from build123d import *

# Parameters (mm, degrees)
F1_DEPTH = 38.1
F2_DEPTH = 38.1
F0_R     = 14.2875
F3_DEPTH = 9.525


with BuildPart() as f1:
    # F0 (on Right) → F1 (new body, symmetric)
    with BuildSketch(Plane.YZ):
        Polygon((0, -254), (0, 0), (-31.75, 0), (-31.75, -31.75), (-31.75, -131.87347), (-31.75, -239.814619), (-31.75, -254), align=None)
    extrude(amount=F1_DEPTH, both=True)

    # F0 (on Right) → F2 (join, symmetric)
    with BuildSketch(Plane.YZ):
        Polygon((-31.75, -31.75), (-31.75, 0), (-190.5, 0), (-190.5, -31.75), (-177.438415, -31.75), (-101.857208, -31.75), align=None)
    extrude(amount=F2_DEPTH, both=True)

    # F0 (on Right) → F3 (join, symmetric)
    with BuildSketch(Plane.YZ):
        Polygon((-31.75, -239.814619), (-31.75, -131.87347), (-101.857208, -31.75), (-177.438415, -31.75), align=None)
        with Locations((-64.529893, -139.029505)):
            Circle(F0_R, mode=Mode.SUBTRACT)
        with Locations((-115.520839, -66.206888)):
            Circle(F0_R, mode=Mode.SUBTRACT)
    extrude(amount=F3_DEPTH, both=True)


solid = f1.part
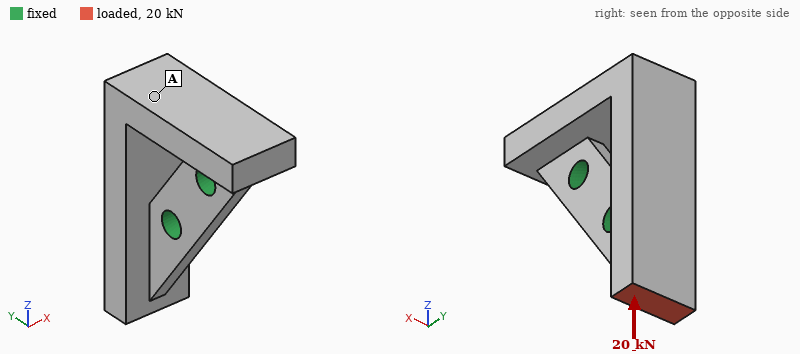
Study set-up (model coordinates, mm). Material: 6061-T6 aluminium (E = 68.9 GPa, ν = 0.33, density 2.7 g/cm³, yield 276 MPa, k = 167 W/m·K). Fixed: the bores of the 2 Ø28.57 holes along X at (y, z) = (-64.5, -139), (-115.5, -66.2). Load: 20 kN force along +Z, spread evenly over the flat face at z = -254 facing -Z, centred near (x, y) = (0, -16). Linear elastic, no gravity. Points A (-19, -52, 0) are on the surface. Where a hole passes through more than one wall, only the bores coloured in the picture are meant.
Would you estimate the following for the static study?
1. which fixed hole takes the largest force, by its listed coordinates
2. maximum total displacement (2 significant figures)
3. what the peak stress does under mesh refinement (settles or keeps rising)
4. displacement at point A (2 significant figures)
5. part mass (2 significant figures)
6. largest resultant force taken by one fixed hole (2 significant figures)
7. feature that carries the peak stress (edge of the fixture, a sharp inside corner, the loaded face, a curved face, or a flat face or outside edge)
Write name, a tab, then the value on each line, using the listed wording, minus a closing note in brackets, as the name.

which fixed hole takes the largest force, by its listed coordinates	(-64.5, -139)
maximum total displacement	0.11 mm
what the peak stress does under mesh refinement	keeps rising
displacement at point A	0.036 mm
part mass	3.2 kg
largest resultant force taken by one fixed hole	19 kN
feature that carries the peak stress	edge of the fixture
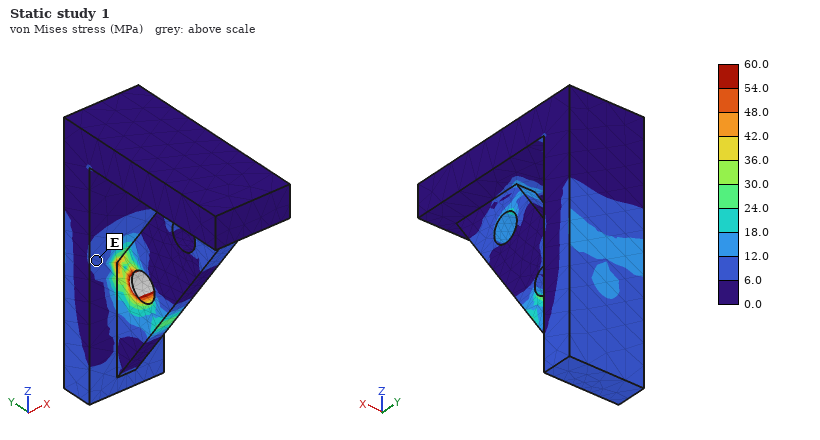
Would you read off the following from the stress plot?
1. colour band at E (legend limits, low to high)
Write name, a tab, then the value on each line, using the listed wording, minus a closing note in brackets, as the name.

colour band at E	6.0 to 12.0 MPa
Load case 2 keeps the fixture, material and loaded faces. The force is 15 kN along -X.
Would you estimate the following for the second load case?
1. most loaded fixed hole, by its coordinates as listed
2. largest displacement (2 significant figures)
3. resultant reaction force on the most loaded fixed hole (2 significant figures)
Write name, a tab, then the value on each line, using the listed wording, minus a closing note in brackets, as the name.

most loaded fixed hole, by its coordinates as listed	(-64.5, -139)
largest displacement	0.65 mm
resultant reaction force on the most loaded fixed hole	23 kN
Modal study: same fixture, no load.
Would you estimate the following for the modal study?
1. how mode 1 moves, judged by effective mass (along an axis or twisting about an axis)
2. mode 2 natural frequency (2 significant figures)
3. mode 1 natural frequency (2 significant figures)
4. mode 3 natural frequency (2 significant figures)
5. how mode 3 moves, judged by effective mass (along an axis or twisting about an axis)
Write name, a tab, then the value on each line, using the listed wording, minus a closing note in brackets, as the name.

how mode 1 moves, judged by effective mass	along X
mode 2 natural frequency	1400 Hz
mode 1 natural frequency	840 Hz
mode 3 natural frequency	1800 Hz
how mode 3 moves, judged by effective mass	along Z
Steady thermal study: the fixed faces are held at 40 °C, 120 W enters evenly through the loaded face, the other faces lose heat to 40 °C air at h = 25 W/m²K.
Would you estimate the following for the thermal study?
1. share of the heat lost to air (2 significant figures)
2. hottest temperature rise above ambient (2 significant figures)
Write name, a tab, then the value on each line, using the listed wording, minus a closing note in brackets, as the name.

share of the heat lost to air	19 %
hottest temperature rise above ambient	36 K
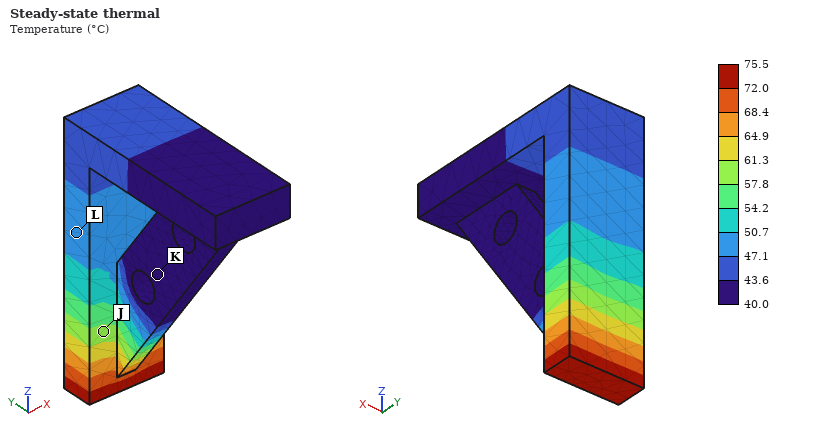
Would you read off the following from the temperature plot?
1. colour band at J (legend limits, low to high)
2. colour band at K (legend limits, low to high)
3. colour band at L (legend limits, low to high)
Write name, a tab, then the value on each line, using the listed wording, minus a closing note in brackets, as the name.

colour band at J	57.8 to 61.3 °C
colour band at K	40.0 to 43.6 °C
colour band at L	47.1 to 50.7 °C
